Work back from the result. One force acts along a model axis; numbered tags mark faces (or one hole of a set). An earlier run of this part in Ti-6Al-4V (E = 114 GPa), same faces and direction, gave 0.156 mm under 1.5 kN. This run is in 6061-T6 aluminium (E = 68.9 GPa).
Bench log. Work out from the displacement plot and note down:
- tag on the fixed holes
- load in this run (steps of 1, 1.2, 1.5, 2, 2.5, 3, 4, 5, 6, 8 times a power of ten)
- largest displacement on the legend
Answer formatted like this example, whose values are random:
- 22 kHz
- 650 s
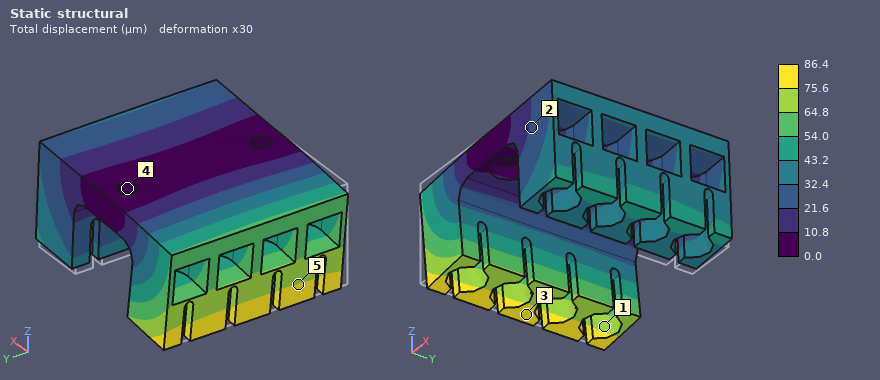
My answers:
- 4
- 500 N
- 86.4 µm
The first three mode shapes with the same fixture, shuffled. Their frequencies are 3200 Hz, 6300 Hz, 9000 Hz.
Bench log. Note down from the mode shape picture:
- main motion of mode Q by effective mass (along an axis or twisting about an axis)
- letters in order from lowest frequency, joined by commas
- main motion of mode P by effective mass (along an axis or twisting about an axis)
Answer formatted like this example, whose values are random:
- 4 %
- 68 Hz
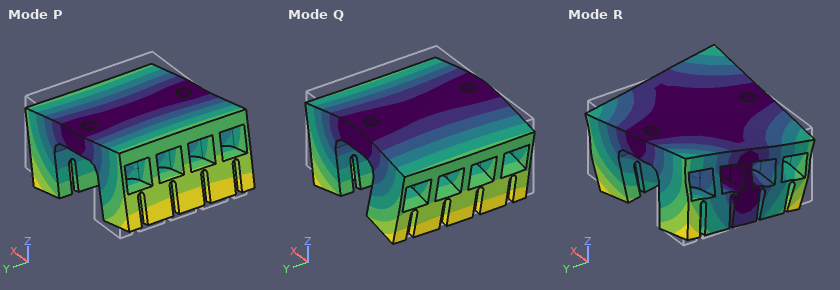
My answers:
- along Z
- P, Q, R
- along X
